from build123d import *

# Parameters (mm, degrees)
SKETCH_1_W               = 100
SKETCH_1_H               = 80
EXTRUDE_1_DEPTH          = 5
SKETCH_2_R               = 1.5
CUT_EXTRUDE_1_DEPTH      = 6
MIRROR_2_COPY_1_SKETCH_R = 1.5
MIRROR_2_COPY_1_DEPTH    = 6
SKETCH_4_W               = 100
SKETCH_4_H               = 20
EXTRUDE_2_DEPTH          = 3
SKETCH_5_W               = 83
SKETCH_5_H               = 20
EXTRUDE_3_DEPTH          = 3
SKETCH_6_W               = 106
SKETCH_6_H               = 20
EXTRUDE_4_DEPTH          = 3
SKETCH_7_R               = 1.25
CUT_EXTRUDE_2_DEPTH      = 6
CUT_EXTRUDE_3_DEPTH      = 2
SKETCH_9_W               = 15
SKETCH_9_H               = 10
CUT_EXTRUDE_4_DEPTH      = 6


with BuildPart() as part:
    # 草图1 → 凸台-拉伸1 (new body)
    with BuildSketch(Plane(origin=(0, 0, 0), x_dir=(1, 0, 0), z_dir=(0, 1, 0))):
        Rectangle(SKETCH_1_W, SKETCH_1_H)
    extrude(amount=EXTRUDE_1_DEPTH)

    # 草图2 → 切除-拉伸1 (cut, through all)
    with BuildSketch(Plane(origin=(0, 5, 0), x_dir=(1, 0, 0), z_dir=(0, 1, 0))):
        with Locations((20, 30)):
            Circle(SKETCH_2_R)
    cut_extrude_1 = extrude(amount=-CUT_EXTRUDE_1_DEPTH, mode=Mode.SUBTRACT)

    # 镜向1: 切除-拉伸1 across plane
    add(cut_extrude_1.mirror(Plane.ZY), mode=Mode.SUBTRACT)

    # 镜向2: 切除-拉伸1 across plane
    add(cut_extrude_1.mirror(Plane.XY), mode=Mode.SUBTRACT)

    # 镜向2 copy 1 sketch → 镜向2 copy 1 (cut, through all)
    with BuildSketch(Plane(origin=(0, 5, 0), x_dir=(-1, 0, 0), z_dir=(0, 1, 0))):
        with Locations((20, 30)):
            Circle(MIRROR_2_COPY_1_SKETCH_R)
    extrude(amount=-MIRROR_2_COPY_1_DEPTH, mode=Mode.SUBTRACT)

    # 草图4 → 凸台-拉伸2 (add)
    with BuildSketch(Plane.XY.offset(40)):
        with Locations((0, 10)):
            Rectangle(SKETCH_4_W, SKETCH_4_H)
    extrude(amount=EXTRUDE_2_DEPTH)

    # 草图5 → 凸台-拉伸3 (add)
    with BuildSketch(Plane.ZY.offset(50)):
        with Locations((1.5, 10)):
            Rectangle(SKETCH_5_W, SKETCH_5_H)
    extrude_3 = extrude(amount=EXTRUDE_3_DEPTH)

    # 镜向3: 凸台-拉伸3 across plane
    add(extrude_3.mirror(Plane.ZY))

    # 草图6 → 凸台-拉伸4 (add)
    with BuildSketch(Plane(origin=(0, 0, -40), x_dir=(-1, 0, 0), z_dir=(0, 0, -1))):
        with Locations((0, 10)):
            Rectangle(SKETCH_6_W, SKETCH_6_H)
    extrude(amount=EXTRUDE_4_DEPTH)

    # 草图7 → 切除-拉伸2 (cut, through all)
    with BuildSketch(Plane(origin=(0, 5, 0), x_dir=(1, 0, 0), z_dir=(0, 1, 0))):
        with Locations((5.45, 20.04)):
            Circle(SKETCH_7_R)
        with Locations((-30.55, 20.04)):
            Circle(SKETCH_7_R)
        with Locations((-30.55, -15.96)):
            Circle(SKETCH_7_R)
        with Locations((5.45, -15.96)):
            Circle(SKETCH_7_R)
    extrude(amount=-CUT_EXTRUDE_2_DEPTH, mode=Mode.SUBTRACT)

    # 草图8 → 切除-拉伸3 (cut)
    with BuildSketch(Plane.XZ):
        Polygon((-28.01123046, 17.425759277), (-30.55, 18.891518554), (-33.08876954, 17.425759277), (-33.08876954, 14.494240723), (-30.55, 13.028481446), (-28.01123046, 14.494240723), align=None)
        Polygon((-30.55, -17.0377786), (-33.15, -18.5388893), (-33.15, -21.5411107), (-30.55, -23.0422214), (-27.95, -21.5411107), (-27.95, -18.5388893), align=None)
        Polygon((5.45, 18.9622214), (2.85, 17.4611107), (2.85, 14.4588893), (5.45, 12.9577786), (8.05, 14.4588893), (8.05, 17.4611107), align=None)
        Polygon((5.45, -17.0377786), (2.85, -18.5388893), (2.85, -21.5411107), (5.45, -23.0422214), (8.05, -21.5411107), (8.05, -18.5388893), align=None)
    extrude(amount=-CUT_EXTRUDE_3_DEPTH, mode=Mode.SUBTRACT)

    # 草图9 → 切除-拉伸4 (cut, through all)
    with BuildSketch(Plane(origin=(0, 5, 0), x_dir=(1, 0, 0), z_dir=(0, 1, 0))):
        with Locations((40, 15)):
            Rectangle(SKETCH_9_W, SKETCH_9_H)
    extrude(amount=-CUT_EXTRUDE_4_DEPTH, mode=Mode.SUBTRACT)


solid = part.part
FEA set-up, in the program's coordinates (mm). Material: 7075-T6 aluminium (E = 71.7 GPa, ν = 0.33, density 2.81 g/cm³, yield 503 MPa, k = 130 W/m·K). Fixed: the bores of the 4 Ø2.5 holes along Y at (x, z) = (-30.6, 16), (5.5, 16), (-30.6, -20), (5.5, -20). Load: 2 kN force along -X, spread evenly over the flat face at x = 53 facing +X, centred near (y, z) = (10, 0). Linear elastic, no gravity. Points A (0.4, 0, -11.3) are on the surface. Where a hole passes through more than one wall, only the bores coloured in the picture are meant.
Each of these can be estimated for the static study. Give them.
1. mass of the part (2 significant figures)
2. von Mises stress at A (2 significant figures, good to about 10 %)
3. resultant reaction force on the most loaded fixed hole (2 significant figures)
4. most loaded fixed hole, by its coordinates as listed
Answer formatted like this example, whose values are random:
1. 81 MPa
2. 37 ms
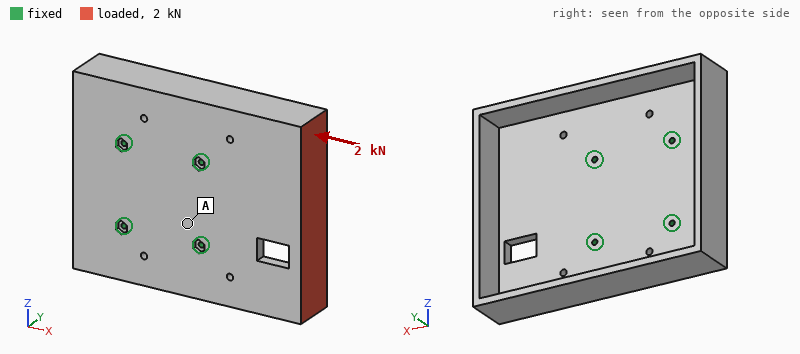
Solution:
1. 170 g
2. 6.1 MPa
3. 730 N
4. (5.5, 16)
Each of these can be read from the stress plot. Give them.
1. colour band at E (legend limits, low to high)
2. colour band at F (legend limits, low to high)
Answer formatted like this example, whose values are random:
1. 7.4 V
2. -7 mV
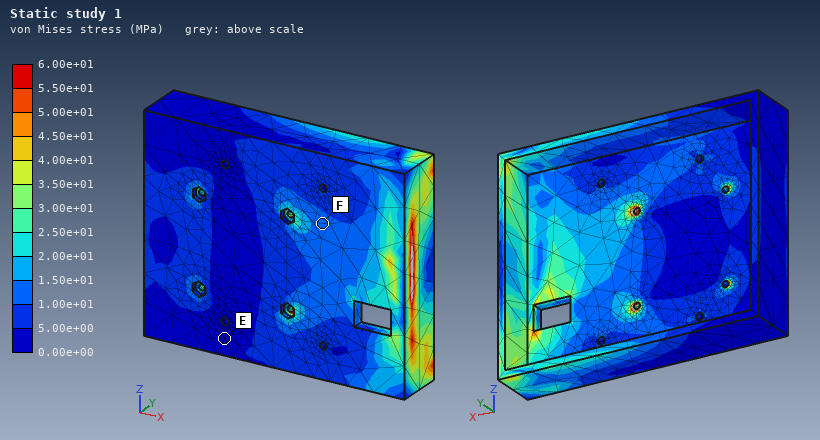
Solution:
1. 0.00e+00 to 5.00e+00 MPa
2. 1.00e+01 to 1.50e+01 MPa
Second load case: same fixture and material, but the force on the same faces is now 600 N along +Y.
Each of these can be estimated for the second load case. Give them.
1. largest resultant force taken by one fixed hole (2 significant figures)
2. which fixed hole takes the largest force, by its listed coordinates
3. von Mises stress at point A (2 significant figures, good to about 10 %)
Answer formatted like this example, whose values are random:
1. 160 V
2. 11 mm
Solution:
1. 700 N
2. (5.5, 16)
3. 24 MPa
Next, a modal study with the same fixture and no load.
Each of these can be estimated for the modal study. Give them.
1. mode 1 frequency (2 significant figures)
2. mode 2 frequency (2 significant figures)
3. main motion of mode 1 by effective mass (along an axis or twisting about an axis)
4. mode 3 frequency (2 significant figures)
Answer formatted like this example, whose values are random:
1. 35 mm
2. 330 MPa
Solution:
1. 1500 Hz
2. 1800 Hz
3. along Y
4. 3000 Hz
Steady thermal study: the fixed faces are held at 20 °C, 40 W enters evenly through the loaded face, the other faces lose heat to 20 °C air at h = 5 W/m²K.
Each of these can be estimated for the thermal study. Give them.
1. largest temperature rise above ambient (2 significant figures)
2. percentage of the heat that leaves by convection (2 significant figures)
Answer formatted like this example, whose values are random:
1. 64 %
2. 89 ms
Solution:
1. 46 K
2. 5.2 %
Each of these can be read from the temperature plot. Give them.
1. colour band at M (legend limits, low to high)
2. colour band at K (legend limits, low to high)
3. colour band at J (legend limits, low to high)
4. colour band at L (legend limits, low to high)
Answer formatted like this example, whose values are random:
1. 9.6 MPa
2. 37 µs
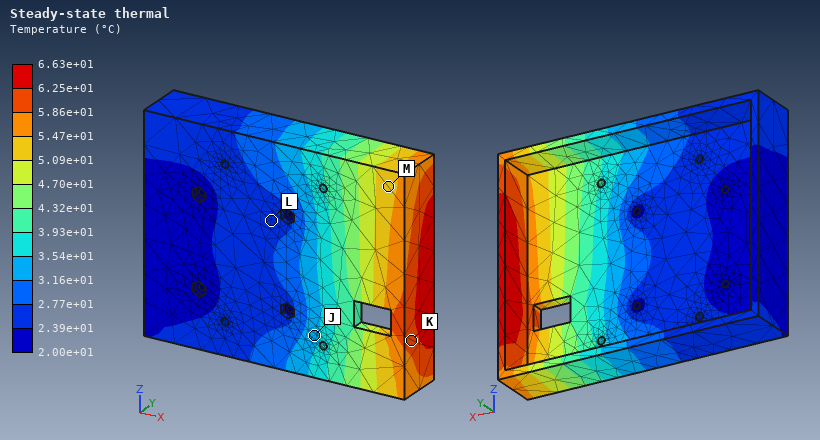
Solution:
1. 5.09e+01 to 5.47e+01 °C
2. 5.86e+01 to 6.25e+01 °C
3. 3.16e+01 to 3.54e+01 °C
4. 2.39e+01 to 2.77e+01 °C
